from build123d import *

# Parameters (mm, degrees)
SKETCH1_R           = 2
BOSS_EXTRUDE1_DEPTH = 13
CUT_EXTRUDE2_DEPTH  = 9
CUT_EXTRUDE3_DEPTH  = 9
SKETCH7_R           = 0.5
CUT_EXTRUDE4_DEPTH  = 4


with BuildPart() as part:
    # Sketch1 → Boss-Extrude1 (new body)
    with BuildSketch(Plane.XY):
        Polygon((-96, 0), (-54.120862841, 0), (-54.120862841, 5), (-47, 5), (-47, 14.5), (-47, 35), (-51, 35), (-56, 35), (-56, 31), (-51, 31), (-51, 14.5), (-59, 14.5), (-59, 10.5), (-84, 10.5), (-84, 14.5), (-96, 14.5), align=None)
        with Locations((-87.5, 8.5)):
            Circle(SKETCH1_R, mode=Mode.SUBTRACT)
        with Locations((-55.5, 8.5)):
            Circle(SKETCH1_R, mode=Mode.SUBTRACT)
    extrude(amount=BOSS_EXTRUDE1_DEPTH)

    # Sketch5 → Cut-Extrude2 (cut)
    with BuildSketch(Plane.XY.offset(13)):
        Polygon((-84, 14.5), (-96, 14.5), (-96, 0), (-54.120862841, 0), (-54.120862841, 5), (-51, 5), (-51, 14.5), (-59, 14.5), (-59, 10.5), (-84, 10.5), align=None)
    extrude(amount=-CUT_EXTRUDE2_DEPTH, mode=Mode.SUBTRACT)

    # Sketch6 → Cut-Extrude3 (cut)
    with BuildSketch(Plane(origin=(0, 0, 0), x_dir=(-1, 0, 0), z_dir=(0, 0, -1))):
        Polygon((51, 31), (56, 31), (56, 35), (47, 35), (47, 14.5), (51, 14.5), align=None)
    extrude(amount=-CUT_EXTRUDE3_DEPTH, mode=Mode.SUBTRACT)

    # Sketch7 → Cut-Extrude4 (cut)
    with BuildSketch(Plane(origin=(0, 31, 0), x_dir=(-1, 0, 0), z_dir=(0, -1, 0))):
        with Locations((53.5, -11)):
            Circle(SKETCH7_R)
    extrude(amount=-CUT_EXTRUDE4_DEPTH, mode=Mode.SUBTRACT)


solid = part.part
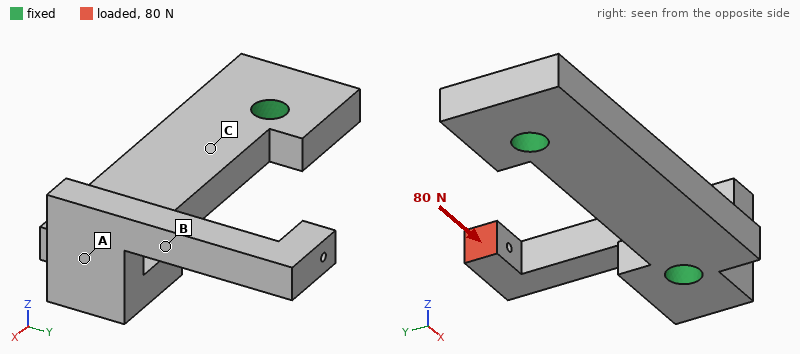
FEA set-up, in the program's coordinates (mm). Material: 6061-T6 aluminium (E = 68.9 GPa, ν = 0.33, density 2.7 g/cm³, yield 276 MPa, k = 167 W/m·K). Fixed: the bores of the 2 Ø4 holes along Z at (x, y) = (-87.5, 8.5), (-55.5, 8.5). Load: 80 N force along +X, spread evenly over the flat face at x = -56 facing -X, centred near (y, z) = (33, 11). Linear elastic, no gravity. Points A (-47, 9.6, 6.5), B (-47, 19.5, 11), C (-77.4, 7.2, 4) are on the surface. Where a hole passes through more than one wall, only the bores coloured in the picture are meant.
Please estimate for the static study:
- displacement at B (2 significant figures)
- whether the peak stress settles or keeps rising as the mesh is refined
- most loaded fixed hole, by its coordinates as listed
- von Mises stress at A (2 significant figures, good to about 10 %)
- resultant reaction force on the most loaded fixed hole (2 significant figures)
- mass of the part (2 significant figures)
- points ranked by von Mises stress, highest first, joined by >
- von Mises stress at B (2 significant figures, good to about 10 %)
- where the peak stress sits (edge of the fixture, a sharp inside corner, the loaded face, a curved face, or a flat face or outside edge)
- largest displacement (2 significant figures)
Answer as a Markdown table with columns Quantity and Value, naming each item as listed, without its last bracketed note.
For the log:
| Quantity | Value |
|---|---|
| displacement at B | 0.084 mm |
| whether the peak stress settles or keeps rising as the mesh is refined | keeps rising |
| most loaded fixed hole, by its coordinates as listed | (-55.5, 8.5) |
| von Mises stress at A | 67 MPa |
| resultant reaction force on the most loaded fixed hole | 99 N |
| mass of the part | 8.0 g |
| points ranked by von Mises stress, highest first, joined by > | B > A > C |
| von Mises stress at B | 100 MPa |
| where the peak stress sits | a sharp inside corner |
| largest displacement | 0.33 mm |
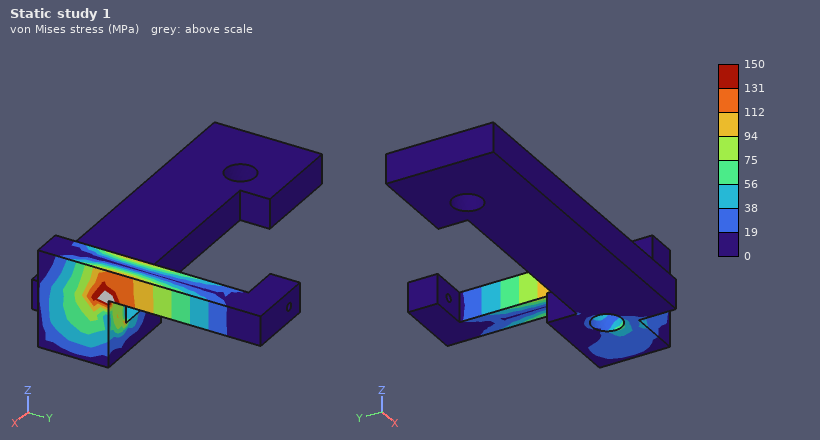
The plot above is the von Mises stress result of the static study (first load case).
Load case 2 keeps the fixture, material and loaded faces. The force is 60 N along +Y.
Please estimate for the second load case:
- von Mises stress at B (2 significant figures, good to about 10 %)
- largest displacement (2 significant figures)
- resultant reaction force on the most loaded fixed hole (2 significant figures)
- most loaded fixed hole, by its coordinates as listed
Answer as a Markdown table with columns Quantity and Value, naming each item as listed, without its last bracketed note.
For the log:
| Quantity | Value |
|---|---|
| von Mises stress at B | 36 MPa |
| largest displacement | 0.12 mm |
| resultant reaction force on the most loaded fixed hole | 60 N |
| most loaded fixed hole, by its coordinates as listed | (-55.5, 8.5) |
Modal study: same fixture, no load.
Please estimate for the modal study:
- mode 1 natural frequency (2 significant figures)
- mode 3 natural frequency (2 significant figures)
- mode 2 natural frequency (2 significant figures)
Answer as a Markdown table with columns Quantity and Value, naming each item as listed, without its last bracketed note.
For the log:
| Quantity | Value |
|---|---|
| mode 1 natural frequency | 3500 Hz |
| mode 3 natural frequency | 11 kHz |
| mode 2 natural frequency | 4000 Hz |
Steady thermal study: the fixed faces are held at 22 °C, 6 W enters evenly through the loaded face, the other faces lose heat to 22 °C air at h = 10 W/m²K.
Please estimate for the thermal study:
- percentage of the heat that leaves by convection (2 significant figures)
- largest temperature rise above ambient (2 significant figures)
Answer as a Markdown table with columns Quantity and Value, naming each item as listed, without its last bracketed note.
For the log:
| Quantity | Value |
|---|---|
| percentage of the heat that leaves by convection | 3.6 % |
| largest temperature rise above ambient | 69 K |
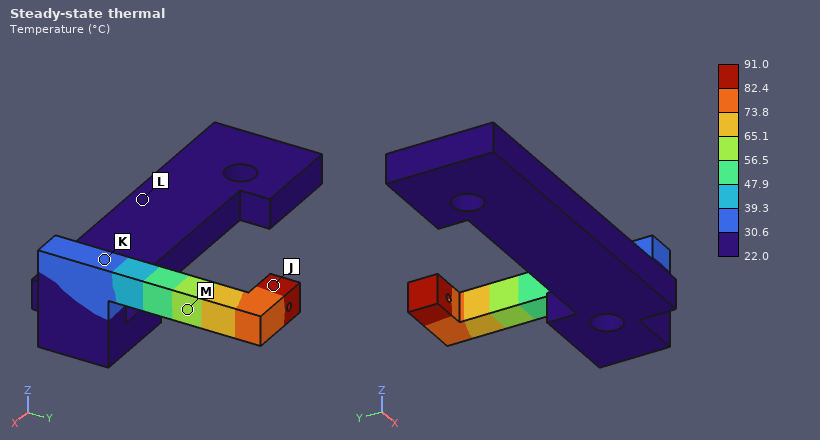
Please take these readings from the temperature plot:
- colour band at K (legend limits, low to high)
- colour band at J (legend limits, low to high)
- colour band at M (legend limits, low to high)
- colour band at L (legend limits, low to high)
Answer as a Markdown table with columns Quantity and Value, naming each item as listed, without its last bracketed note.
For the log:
| Quantity | Value |
|---|---|
| colour band at K | 30.6 to 39.3 °C |
| colour band at J | 82.4 to 91.0 °C |
| colour band at M | 56.5 to 65.1 °C |
| colour band at L | 22.0 to 30.6 °C |
